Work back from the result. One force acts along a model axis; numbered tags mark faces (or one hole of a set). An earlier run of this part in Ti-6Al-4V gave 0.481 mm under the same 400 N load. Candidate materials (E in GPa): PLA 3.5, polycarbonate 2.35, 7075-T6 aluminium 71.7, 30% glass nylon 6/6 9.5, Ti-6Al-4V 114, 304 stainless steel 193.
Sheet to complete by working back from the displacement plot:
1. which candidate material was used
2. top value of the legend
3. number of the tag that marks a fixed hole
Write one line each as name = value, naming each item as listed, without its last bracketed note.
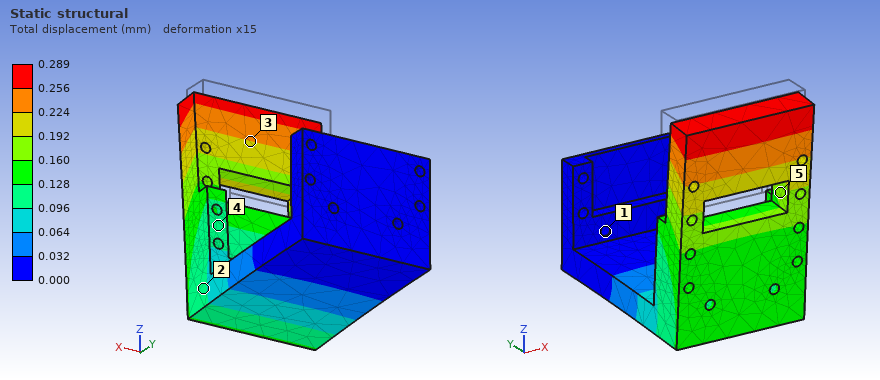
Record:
which candidate material was used = 304 stainless steel
top value of the legend = 0.289 mm
number of the tag that marks a fixed hole = 1
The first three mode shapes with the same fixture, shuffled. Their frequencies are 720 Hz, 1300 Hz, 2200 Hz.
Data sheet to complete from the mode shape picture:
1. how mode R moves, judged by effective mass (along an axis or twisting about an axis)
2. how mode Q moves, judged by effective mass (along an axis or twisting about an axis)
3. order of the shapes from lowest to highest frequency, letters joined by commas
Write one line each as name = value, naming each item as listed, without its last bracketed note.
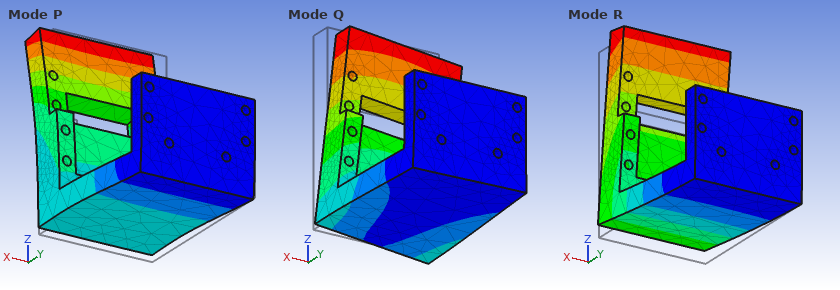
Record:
how mode R moves, judged by effective mass = along Z
how mode Q moves, judged by effective mass = along X
order of the shapes from lowest to highest frequency, letters joined by commas = R, Q, P
